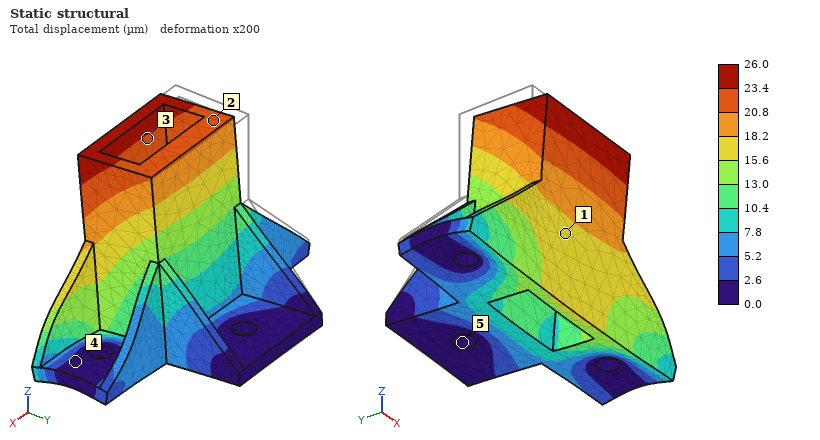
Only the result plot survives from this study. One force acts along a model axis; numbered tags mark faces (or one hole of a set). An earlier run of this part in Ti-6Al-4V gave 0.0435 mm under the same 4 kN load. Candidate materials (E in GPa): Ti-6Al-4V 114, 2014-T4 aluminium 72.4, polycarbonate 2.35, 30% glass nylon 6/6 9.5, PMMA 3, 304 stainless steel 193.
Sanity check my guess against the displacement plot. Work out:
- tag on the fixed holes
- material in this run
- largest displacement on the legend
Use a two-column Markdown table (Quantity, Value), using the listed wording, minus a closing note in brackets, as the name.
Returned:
| Quantity | Value |
|---|---|
| tag on the fixed holes | 5 |
| material in this run | 304 stainless steel |
| largest displacement on the legend | 26.0 µm |
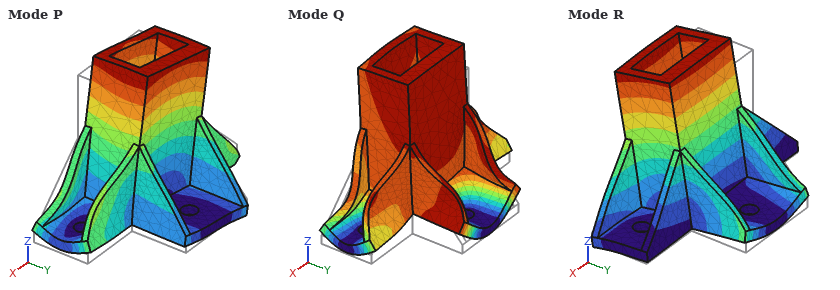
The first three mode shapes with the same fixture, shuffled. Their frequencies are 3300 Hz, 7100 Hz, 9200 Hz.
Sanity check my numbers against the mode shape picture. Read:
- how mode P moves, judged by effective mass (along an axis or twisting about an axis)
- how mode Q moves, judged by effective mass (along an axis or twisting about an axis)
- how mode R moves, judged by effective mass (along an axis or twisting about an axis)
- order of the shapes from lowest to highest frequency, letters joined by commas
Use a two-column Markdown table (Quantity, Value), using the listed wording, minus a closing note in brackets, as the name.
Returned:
| Quantity | Value |
|---|---|
| how mode P moves, judged by effective mass | along X |
| how mode Q moves, judged by effective mass | along Z |
| how mode R moves, judged by effective mass | along Y |
| order of the shapes from lowest to highest frequency, letters joined by commas | R, P, Q |
